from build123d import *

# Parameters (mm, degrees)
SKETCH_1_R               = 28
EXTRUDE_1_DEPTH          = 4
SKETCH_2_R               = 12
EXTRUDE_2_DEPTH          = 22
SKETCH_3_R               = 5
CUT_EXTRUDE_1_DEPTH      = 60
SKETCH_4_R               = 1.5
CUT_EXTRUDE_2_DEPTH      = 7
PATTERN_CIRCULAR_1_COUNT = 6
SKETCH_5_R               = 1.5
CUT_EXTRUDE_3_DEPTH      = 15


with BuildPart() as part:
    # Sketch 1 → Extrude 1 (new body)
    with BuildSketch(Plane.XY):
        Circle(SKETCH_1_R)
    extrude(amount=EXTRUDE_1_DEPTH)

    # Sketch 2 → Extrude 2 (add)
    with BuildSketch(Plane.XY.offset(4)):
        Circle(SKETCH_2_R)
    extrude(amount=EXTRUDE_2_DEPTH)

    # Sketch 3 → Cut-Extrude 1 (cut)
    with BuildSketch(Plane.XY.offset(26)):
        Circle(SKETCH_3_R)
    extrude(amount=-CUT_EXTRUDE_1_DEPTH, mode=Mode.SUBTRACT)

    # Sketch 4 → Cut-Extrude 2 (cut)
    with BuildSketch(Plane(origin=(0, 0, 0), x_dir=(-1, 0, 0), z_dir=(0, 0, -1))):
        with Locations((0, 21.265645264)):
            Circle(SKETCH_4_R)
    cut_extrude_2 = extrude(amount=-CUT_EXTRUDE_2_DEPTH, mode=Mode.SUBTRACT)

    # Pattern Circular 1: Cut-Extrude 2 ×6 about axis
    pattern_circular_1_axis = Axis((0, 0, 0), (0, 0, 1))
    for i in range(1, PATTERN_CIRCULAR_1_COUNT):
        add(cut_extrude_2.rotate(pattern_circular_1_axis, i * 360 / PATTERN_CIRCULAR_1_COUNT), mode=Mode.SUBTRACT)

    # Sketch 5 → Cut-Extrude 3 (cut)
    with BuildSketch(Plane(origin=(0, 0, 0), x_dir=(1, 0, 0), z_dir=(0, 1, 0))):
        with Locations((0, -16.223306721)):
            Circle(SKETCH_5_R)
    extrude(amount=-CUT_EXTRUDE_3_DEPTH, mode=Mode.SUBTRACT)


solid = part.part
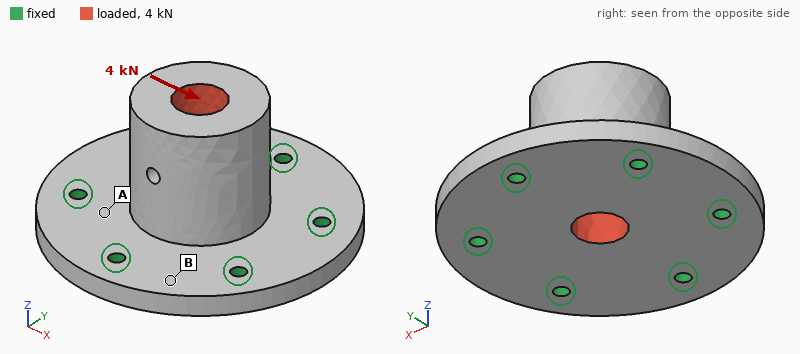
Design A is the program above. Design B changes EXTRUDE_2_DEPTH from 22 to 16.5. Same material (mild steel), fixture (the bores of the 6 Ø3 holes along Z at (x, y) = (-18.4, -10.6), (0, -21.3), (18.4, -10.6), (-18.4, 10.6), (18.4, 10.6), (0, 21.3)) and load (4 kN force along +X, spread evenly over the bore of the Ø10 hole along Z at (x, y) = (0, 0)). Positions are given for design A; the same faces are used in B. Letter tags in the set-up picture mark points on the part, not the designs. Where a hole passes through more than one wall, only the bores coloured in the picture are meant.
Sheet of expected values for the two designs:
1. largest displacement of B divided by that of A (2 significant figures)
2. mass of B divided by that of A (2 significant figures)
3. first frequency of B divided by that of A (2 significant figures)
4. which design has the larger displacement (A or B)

0.61
0.88
1.4
A
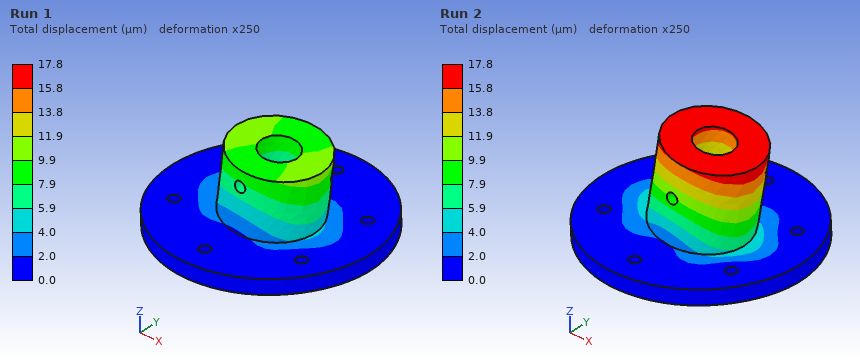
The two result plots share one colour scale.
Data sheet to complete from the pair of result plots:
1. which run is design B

Run 1
